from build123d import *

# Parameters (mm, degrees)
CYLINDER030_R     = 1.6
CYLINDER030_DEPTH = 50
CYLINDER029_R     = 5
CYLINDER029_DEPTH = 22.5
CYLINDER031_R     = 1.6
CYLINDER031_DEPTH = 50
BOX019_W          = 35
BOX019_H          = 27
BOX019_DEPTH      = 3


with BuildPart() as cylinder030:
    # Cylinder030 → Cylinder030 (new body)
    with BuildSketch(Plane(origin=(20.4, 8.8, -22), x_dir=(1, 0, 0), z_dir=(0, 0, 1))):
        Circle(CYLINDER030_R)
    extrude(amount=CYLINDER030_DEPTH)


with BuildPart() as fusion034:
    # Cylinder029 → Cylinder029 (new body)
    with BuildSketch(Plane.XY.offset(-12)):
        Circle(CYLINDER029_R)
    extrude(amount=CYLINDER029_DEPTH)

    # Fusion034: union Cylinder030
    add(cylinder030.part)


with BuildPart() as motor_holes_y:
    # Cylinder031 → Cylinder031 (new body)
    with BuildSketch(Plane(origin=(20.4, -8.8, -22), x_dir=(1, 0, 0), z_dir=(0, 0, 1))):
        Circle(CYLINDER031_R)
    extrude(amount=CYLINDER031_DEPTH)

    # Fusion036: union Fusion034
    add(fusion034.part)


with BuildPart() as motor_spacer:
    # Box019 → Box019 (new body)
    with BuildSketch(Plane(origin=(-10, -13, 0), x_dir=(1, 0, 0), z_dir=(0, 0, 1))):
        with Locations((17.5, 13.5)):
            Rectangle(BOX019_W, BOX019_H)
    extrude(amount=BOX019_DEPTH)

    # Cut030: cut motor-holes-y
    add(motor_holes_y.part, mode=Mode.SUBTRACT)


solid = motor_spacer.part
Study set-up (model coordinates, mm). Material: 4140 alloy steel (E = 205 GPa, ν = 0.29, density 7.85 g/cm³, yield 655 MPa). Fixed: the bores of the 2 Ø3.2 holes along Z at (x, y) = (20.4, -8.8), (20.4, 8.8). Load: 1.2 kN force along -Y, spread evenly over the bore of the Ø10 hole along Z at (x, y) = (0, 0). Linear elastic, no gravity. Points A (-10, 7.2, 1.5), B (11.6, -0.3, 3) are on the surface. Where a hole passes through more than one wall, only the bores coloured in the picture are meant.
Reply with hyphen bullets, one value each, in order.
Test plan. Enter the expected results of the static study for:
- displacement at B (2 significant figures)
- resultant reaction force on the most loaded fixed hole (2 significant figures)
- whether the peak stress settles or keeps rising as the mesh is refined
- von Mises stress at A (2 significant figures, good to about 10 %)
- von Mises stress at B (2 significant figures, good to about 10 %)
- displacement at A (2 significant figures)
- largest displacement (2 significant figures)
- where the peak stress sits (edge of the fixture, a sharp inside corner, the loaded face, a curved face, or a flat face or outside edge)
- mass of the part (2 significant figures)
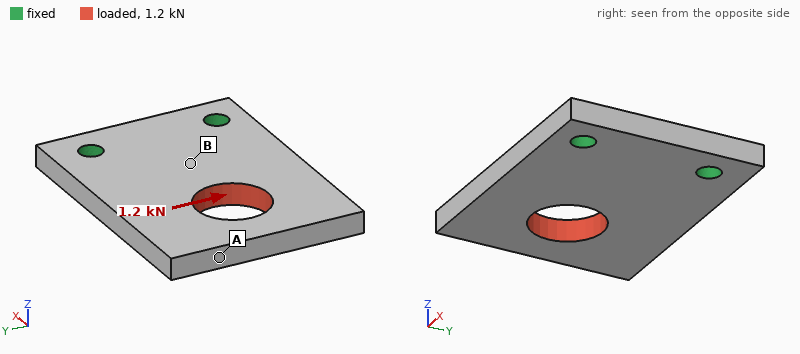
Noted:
- 3.0 µm
- 1.4 kN
- keeps rising
- 19 MPa
- 50 MPa
- 15 µm
- 15 µm
- edge of the fixture
- 20 g
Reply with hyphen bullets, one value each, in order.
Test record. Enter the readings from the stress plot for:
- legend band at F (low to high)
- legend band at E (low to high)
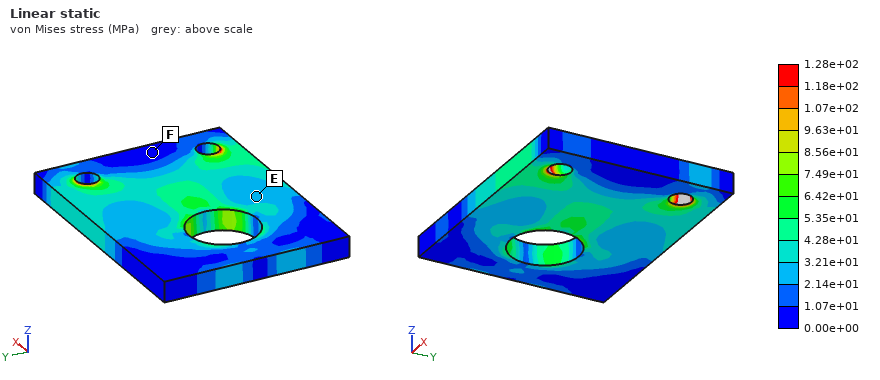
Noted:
- 0.00e+00 to 1.07e+01 MPa
- 2.14e+01 to 3.21e+01 MPa
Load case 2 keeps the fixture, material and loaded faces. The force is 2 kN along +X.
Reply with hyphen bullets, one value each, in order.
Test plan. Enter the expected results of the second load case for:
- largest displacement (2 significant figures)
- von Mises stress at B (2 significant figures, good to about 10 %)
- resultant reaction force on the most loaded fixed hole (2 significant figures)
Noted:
- 5.7 µm
- 18 MPa
- 1.0 kN
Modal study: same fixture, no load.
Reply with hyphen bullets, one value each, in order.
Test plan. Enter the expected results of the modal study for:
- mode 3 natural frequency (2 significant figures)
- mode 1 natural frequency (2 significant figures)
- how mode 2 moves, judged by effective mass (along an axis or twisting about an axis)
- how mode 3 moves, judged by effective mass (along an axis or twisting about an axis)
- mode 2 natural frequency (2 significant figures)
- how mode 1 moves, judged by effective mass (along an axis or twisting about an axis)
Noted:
- 15 kHz
- 2800 Hz
- twisting about X
- along Z
- 6700 Hz
- along Z
